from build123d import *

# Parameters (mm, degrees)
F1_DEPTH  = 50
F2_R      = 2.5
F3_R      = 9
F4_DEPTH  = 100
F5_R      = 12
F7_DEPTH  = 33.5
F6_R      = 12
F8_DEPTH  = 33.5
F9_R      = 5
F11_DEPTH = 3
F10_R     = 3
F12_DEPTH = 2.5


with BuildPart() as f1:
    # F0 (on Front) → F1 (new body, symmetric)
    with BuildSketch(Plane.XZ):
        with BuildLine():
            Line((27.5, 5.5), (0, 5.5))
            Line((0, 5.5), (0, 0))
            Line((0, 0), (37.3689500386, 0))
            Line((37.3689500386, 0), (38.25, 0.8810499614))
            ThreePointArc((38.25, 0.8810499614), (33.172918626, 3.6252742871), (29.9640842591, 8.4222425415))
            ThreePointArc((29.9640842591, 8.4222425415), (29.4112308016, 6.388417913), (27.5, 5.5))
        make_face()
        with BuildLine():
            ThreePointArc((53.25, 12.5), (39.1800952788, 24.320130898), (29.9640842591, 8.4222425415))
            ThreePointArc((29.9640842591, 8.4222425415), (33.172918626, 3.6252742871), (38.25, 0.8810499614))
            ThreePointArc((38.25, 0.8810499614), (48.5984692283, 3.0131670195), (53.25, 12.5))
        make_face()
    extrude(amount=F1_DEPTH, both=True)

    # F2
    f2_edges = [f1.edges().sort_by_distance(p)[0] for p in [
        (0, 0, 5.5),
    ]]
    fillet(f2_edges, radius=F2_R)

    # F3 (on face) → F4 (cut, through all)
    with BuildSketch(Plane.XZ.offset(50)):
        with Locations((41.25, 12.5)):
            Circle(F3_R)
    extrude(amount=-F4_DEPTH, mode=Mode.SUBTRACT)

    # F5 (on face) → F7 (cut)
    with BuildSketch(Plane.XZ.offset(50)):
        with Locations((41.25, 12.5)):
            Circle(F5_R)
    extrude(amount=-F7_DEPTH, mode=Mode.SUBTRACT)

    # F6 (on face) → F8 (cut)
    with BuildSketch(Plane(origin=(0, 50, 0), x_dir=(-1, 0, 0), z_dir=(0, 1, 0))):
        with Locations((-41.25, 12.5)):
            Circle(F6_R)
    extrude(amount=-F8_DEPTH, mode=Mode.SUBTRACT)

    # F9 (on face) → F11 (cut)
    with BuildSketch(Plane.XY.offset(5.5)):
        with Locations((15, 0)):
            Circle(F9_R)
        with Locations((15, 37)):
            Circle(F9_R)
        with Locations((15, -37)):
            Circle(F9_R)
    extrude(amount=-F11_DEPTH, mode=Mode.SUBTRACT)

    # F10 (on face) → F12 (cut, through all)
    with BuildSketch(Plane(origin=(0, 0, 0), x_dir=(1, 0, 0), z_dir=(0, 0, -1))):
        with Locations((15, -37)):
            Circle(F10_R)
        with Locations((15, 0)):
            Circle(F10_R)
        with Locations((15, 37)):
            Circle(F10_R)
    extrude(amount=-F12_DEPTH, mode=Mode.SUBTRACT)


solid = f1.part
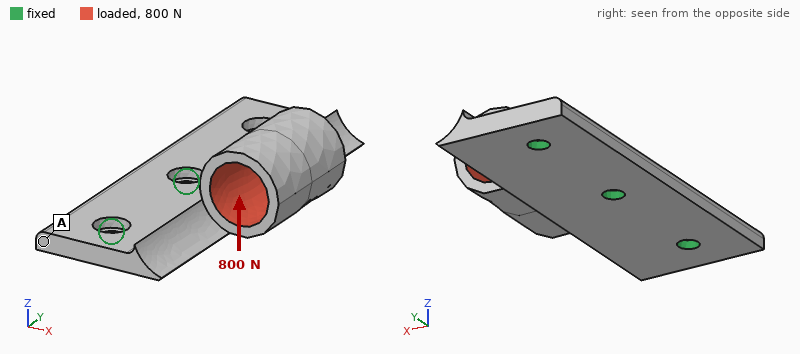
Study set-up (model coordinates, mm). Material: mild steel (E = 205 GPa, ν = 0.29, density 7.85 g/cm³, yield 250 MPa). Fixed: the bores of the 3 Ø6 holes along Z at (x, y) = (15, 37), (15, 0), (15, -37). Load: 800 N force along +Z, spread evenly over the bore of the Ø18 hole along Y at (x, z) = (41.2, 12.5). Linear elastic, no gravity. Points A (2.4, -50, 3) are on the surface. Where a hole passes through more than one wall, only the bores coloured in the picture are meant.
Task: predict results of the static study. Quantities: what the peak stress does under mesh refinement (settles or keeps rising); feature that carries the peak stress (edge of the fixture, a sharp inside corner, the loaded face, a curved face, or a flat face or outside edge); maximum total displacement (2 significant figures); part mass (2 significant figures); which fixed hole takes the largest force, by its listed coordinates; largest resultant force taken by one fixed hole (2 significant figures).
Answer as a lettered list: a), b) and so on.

a) keeps rising
b) edge of the fixture
c) 0.10 mm
d) 200 g
e) (15, 0)
f) 580 N
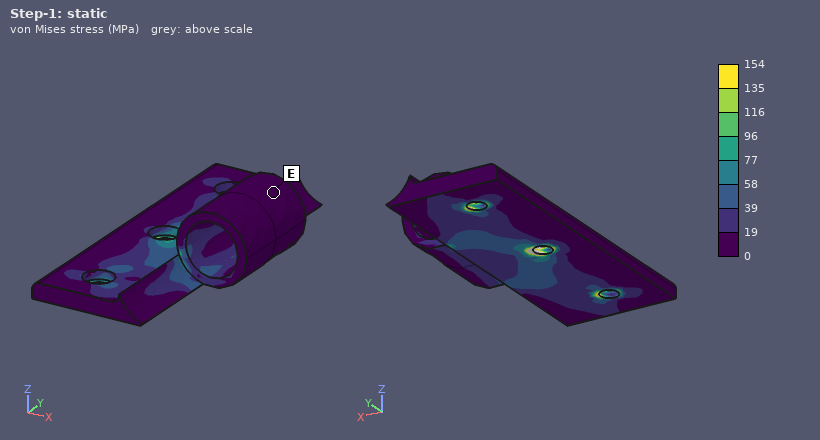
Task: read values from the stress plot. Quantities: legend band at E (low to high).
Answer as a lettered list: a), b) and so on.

a) 0 to 19 MPa
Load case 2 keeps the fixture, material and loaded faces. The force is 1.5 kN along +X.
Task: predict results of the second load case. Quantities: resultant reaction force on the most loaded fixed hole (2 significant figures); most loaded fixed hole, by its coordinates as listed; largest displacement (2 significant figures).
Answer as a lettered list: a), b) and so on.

a) 960 N
b) (15, 0)
c) 0.11 mm
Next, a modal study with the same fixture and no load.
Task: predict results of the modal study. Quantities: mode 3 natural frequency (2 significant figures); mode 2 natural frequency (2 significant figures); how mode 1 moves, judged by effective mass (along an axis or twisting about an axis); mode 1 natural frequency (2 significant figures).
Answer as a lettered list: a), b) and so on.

a) 7000 Hz
b) 5800 Hz
c) along Z
d) 2000 Hz
